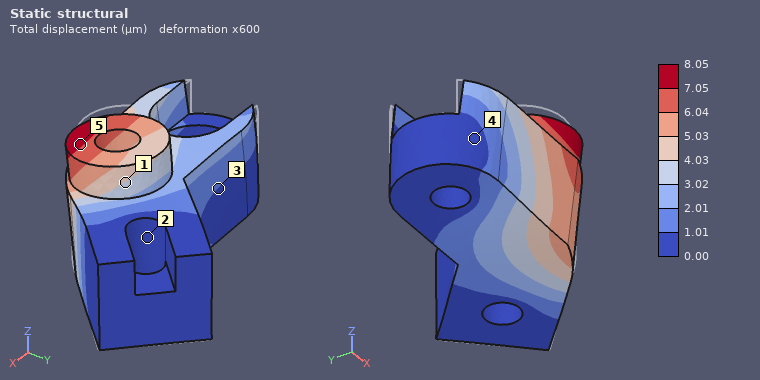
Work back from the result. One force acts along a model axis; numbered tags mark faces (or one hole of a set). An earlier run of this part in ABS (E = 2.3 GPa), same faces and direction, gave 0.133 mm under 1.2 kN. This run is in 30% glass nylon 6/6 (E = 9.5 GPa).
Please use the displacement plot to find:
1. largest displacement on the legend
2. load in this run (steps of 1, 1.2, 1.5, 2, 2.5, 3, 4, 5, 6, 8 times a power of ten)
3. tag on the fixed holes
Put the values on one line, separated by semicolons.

8.05 µm; 300 N; 2
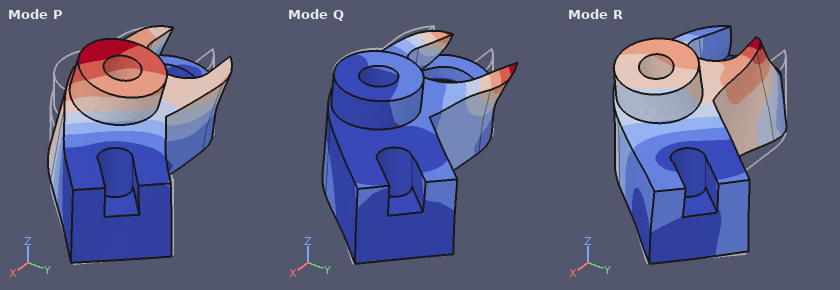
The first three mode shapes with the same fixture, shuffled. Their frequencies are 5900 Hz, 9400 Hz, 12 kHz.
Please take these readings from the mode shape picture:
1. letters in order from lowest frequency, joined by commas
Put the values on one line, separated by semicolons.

P, R, Q
